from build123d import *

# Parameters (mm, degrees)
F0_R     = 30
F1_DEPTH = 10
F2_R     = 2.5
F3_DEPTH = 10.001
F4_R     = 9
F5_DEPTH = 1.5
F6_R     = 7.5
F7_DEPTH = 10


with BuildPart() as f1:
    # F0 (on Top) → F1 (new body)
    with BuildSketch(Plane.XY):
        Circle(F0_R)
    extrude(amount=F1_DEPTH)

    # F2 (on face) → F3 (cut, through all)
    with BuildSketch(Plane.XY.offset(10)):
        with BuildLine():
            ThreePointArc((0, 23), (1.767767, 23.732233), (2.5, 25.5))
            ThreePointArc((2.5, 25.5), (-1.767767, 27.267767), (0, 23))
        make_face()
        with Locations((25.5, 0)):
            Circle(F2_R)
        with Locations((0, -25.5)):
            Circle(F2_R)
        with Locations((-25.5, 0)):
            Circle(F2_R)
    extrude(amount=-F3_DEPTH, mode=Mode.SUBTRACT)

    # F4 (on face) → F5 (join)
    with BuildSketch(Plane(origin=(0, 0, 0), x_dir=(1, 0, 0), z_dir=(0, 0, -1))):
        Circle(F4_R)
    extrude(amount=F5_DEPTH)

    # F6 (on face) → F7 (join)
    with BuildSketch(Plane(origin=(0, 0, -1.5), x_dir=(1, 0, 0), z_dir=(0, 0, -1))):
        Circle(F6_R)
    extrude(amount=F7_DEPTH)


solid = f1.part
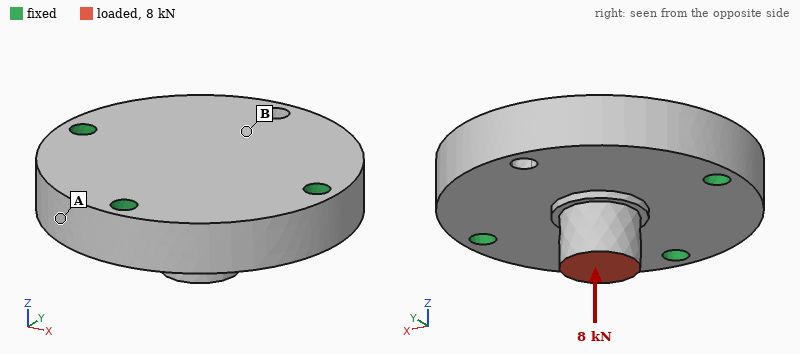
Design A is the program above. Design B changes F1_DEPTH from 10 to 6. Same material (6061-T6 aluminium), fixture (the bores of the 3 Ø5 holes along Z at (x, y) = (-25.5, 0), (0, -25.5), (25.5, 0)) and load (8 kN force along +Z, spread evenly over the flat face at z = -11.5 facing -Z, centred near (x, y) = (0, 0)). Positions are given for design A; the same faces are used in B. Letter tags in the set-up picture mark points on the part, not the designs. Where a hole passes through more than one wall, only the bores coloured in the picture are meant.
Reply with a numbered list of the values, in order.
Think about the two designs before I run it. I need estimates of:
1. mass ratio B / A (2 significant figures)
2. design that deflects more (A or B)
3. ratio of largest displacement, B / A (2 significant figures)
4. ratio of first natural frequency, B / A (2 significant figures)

1. 0.63
2. B
3. 3.4
4. 0.68
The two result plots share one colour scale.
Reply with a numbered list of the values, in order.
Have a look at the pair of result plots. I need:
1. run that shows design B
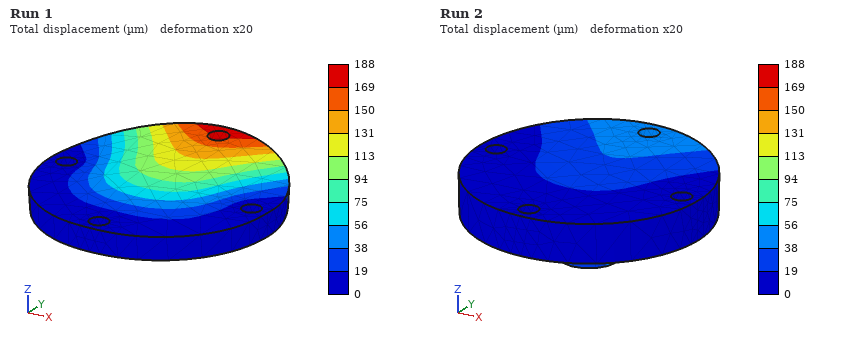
1. Run 1
